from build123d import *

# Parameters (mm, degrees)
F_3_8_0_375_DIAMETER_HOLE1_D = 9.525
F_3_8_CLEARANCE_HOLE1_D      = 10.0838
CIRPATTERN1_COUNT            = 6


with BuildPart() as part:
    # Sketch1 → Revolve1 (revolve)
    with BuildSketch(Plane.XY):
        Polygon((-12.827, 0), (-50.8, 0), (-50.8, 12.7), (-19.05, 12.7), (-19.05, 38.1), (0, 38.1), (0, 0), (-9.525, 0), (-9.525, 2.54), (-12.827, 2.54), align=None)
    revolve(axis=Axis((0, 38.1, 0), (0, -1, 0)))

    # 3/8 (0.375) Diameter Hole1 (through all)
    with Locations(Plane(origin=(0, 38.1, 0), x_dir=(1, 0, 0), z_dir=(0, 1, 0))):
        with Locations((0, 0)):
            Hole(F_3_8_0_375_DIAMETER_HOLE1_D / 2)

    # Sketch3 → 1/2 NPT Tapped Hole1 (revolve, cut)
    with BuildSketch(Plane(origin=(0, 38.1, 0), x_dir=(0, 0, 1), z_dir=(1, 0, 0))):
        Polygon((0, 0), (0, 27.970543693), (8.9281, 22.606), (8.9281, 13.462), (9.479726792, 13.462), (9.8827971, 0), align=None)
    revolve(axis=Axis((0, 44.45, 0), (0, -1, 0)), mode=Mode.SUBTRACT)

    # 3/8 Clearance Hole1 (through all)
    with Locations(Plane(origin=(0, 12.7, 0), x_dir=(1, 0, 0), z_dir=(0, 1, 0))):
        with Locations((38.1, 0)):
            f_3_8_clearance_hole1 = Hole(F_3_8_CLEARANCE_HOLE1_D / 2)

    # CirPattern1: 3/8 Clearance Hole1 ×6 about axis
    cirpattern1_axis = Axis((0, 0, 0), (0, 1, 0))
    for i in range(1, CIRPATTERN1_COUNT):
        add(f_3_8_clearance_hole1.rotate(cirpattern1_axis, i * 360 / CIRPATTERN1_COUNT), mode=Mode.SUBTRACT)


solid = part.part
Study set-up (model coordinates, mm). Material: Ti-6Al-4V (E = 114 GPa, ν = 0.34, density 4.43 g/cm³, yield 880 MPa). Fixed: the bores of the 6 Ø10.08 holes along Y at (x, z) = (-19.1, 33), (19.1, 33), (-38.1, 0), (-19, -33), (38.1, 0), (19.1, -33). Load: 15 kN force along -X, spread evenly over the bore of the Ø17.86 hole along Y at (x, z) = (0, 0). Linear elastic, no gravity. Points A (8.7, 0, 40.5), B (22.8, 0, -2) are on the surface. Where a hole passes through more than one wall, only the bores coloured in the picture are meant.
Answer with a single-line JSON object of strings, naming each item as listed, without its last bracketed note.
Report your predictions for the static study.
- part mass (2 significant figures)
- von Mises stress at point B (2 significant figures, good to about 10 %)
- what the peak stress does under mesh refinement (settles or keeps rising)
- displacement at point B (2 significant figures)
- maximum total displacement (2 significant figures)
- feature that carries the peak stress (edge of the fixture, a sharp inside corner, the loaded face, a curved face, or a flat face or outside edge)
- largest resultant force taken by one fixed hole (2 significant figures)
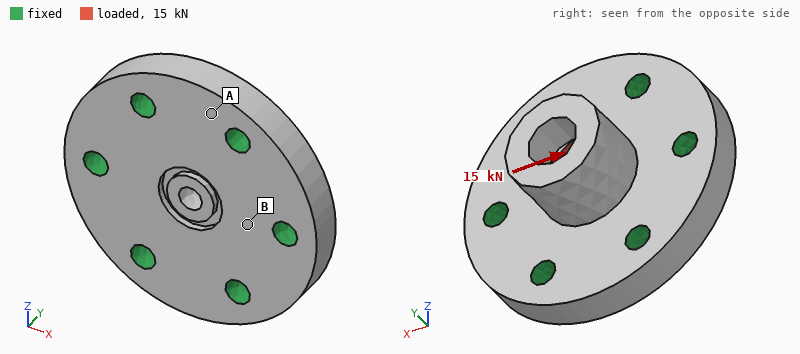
{"part mass": "520 g", "von Mises stress at point B": "10.0 MPa", "what the peak stress does under mesh refinement": "keeps rising", "displacement at point B": "3.6 µm", "maximum total displacement": "15 µm", "feature that carries the peak stress": "edge of the fixture", "largest resultant force taken by one fixed hole": "4.5 kN"}
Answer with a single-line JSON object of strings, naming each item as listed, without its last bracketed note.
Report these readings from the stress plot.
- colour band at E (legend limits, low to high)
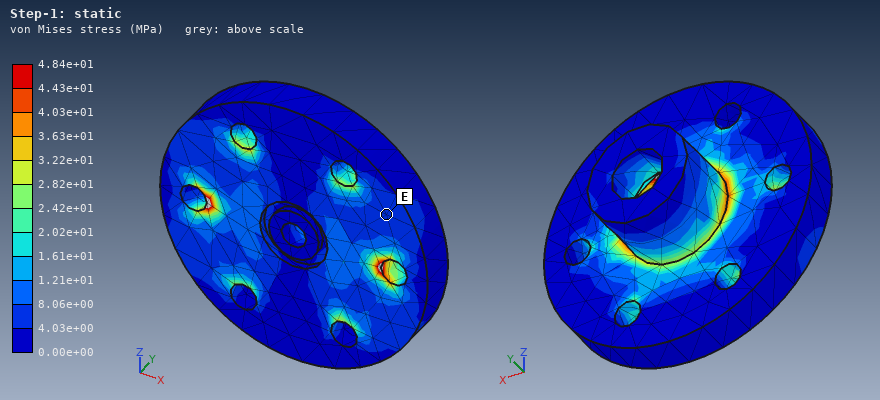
{"colour band at E": "4.03e+00 to 8.06e+00 MPa"}
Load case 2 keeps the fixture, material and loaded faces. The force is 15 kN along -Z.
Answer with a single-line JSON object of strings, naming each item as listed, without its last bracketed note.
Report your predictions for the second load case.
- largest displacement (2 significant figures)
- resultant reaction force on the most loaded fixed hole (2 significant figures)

{"largest displacement": "15 µm", "resultant reaction force on the most loaded fixed hole": "4.0 kN"}
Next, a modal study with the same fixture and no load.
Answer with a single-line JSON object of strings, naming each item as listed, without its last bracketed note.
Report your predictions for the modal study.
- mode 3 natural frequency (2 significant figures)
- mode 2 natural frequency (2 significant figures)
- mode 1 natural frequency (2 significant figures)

{"mode 3 natural frequency": "14 kHz", "mode 2 natural frequency": "14 kHz", "mode 1 natural frequency": "14 kHz"}
